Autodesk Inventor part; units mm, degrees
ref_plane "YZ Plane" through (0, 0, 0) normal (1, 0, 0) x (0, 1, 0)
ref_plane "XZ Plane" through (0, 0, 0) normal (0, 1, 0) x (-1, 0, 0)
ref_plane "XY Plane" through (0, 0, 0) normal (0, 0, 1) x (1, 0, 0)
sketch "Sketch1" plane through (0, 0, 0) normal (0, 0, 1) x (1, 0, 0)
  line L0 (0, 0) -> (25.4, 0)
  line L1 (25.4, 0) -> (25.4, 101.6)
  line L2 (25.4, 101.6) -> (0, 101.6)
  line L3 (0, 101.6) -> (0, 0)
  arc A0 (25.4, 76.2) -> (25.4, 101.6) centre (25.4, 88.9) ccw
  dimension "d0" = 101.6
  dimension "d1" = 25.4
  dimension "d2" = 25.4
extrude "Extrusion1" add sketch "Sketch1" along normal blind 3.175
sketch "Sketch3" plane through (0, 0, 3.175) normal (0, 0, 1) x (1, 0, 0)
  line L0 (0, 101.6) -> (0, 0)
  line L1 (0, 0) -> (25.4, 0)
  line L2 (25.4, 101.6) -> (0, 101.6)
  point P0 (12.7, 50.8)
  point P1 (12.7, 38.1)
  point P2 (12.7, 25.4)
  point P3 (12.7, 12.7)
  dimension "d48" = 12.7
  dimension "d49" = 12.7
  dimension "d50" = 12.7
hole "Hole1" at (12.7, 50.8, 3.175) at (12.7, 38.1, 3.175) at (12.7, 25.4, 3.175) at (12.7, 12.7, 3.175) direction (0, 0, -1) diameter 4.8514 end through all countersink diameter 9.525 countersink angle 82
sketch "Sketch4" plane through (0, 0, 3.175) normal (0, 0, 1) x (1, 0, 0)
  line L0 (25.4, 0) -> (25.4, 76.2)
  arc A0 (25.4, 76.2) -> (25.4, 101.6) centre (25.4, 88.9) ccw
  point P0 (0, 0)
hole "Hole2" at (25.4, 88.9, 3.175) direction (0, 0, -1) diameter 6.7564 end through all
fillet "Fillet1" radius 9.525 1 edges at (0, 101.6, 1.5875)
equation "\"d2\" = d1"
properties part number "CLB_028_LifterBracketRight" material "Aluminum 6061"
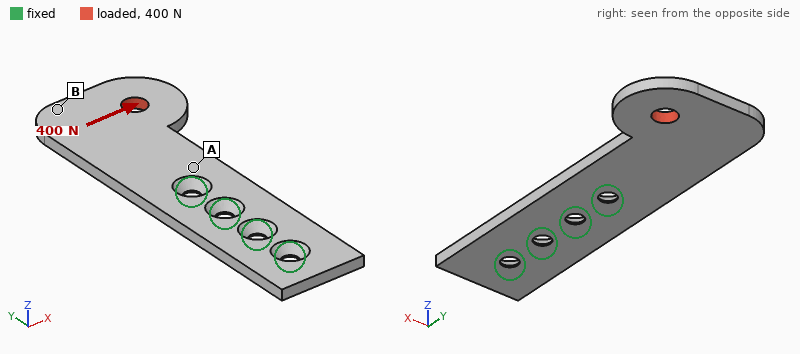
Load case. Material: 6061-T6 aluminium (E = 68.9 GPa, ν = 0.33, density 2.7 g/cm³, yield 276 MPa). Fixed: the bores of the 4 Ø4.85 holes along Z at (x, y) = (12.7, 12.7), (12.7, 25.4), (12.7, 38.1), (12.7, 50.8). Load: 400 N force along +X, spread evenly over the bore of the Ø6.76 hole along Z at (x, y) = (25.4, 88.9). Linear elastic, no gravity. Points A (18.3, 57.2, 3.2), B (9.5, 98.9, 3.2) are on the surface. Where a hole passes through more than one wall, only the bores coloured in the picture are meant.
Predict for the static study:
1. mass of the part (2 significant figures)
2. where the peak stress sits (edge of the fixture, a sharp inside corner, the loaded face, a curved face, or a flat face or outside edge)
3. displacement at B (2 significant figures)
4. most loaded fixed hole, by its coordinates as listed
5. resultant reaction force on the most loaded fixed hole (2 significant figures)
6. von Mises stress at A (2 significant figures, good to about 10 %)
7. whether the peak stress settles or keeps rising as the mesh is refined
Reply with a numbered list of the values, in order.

1. 23 g
2. edge of the fixture
3. 0.091 mm
4. (12.7, 50.8)
5. 900 N
6. 23 MPa
7. keeps rising
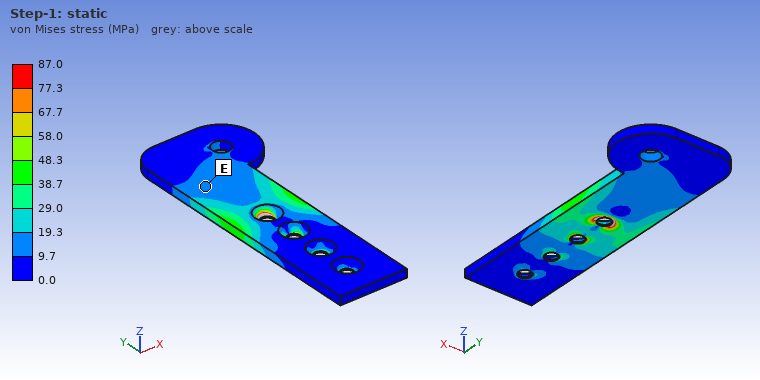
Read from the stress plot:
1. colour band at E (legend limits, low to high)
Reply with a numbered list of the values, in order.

1. 9.7 to 19.3 MPa
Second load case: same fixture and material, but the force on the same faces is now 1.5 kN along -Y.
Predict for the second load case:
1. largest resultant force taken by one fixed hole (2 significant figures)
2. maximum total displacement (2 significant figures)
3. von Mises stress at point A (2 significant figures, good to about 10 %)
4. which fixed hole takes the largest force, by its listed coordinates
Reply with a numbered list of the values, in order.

1. 1.0 kN
2. 0.16 mm
3. 48 MPa
4. (12.7, 50.8)
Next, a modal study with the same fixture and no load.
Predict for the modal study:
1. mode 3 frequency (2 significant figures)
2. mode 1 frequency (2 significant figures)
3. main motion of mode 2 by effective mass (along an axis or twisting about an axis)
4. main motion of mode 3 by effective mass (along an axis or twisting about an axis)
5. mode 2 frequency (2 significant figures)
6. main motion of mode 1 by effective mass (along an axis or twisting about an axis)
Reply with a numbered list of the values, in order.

1. 4100 Hz
2. 780 Hz
3. twisting about Y
4. along X
5. 2100 Hz
6. along Z
